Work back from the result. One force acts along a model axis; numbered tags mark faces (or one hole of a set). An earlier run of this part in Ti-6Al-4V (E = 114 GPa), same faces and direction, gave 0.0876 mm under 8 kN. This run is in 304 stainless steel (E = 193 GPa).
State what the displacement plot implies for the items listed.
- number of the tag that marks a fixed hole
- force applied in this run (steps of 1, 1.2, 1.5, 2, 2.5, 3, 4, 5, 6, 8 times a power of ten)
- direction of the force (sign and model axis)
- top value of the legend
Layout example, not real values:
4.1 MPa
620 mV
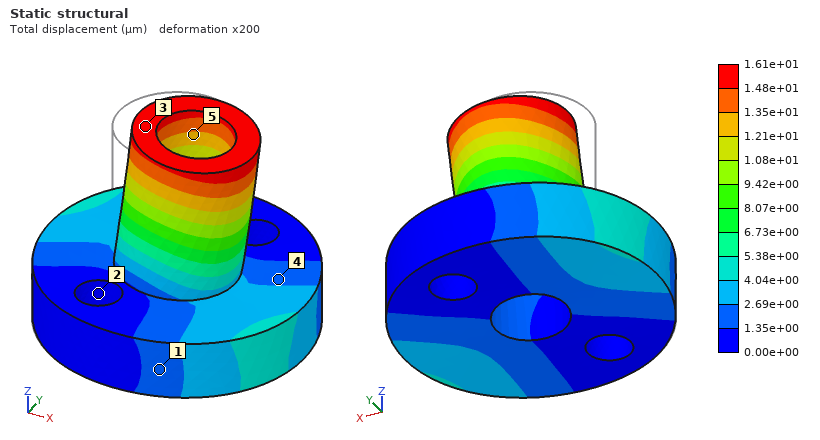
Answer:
2
2.5 kN
+X
1.61e+01 µm
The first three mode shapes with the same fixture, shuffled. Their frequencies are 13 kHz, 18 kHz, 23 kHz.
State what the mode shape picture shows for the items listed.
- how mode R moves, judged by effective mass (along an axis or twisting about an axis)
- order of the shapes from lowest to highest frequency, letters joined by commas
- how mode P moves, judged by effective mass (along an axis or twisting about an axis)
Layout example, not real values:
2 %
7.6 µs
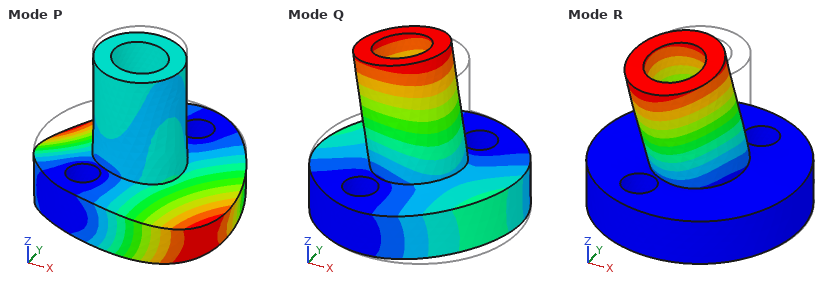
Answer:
along Y
Q, R, P
along Z
